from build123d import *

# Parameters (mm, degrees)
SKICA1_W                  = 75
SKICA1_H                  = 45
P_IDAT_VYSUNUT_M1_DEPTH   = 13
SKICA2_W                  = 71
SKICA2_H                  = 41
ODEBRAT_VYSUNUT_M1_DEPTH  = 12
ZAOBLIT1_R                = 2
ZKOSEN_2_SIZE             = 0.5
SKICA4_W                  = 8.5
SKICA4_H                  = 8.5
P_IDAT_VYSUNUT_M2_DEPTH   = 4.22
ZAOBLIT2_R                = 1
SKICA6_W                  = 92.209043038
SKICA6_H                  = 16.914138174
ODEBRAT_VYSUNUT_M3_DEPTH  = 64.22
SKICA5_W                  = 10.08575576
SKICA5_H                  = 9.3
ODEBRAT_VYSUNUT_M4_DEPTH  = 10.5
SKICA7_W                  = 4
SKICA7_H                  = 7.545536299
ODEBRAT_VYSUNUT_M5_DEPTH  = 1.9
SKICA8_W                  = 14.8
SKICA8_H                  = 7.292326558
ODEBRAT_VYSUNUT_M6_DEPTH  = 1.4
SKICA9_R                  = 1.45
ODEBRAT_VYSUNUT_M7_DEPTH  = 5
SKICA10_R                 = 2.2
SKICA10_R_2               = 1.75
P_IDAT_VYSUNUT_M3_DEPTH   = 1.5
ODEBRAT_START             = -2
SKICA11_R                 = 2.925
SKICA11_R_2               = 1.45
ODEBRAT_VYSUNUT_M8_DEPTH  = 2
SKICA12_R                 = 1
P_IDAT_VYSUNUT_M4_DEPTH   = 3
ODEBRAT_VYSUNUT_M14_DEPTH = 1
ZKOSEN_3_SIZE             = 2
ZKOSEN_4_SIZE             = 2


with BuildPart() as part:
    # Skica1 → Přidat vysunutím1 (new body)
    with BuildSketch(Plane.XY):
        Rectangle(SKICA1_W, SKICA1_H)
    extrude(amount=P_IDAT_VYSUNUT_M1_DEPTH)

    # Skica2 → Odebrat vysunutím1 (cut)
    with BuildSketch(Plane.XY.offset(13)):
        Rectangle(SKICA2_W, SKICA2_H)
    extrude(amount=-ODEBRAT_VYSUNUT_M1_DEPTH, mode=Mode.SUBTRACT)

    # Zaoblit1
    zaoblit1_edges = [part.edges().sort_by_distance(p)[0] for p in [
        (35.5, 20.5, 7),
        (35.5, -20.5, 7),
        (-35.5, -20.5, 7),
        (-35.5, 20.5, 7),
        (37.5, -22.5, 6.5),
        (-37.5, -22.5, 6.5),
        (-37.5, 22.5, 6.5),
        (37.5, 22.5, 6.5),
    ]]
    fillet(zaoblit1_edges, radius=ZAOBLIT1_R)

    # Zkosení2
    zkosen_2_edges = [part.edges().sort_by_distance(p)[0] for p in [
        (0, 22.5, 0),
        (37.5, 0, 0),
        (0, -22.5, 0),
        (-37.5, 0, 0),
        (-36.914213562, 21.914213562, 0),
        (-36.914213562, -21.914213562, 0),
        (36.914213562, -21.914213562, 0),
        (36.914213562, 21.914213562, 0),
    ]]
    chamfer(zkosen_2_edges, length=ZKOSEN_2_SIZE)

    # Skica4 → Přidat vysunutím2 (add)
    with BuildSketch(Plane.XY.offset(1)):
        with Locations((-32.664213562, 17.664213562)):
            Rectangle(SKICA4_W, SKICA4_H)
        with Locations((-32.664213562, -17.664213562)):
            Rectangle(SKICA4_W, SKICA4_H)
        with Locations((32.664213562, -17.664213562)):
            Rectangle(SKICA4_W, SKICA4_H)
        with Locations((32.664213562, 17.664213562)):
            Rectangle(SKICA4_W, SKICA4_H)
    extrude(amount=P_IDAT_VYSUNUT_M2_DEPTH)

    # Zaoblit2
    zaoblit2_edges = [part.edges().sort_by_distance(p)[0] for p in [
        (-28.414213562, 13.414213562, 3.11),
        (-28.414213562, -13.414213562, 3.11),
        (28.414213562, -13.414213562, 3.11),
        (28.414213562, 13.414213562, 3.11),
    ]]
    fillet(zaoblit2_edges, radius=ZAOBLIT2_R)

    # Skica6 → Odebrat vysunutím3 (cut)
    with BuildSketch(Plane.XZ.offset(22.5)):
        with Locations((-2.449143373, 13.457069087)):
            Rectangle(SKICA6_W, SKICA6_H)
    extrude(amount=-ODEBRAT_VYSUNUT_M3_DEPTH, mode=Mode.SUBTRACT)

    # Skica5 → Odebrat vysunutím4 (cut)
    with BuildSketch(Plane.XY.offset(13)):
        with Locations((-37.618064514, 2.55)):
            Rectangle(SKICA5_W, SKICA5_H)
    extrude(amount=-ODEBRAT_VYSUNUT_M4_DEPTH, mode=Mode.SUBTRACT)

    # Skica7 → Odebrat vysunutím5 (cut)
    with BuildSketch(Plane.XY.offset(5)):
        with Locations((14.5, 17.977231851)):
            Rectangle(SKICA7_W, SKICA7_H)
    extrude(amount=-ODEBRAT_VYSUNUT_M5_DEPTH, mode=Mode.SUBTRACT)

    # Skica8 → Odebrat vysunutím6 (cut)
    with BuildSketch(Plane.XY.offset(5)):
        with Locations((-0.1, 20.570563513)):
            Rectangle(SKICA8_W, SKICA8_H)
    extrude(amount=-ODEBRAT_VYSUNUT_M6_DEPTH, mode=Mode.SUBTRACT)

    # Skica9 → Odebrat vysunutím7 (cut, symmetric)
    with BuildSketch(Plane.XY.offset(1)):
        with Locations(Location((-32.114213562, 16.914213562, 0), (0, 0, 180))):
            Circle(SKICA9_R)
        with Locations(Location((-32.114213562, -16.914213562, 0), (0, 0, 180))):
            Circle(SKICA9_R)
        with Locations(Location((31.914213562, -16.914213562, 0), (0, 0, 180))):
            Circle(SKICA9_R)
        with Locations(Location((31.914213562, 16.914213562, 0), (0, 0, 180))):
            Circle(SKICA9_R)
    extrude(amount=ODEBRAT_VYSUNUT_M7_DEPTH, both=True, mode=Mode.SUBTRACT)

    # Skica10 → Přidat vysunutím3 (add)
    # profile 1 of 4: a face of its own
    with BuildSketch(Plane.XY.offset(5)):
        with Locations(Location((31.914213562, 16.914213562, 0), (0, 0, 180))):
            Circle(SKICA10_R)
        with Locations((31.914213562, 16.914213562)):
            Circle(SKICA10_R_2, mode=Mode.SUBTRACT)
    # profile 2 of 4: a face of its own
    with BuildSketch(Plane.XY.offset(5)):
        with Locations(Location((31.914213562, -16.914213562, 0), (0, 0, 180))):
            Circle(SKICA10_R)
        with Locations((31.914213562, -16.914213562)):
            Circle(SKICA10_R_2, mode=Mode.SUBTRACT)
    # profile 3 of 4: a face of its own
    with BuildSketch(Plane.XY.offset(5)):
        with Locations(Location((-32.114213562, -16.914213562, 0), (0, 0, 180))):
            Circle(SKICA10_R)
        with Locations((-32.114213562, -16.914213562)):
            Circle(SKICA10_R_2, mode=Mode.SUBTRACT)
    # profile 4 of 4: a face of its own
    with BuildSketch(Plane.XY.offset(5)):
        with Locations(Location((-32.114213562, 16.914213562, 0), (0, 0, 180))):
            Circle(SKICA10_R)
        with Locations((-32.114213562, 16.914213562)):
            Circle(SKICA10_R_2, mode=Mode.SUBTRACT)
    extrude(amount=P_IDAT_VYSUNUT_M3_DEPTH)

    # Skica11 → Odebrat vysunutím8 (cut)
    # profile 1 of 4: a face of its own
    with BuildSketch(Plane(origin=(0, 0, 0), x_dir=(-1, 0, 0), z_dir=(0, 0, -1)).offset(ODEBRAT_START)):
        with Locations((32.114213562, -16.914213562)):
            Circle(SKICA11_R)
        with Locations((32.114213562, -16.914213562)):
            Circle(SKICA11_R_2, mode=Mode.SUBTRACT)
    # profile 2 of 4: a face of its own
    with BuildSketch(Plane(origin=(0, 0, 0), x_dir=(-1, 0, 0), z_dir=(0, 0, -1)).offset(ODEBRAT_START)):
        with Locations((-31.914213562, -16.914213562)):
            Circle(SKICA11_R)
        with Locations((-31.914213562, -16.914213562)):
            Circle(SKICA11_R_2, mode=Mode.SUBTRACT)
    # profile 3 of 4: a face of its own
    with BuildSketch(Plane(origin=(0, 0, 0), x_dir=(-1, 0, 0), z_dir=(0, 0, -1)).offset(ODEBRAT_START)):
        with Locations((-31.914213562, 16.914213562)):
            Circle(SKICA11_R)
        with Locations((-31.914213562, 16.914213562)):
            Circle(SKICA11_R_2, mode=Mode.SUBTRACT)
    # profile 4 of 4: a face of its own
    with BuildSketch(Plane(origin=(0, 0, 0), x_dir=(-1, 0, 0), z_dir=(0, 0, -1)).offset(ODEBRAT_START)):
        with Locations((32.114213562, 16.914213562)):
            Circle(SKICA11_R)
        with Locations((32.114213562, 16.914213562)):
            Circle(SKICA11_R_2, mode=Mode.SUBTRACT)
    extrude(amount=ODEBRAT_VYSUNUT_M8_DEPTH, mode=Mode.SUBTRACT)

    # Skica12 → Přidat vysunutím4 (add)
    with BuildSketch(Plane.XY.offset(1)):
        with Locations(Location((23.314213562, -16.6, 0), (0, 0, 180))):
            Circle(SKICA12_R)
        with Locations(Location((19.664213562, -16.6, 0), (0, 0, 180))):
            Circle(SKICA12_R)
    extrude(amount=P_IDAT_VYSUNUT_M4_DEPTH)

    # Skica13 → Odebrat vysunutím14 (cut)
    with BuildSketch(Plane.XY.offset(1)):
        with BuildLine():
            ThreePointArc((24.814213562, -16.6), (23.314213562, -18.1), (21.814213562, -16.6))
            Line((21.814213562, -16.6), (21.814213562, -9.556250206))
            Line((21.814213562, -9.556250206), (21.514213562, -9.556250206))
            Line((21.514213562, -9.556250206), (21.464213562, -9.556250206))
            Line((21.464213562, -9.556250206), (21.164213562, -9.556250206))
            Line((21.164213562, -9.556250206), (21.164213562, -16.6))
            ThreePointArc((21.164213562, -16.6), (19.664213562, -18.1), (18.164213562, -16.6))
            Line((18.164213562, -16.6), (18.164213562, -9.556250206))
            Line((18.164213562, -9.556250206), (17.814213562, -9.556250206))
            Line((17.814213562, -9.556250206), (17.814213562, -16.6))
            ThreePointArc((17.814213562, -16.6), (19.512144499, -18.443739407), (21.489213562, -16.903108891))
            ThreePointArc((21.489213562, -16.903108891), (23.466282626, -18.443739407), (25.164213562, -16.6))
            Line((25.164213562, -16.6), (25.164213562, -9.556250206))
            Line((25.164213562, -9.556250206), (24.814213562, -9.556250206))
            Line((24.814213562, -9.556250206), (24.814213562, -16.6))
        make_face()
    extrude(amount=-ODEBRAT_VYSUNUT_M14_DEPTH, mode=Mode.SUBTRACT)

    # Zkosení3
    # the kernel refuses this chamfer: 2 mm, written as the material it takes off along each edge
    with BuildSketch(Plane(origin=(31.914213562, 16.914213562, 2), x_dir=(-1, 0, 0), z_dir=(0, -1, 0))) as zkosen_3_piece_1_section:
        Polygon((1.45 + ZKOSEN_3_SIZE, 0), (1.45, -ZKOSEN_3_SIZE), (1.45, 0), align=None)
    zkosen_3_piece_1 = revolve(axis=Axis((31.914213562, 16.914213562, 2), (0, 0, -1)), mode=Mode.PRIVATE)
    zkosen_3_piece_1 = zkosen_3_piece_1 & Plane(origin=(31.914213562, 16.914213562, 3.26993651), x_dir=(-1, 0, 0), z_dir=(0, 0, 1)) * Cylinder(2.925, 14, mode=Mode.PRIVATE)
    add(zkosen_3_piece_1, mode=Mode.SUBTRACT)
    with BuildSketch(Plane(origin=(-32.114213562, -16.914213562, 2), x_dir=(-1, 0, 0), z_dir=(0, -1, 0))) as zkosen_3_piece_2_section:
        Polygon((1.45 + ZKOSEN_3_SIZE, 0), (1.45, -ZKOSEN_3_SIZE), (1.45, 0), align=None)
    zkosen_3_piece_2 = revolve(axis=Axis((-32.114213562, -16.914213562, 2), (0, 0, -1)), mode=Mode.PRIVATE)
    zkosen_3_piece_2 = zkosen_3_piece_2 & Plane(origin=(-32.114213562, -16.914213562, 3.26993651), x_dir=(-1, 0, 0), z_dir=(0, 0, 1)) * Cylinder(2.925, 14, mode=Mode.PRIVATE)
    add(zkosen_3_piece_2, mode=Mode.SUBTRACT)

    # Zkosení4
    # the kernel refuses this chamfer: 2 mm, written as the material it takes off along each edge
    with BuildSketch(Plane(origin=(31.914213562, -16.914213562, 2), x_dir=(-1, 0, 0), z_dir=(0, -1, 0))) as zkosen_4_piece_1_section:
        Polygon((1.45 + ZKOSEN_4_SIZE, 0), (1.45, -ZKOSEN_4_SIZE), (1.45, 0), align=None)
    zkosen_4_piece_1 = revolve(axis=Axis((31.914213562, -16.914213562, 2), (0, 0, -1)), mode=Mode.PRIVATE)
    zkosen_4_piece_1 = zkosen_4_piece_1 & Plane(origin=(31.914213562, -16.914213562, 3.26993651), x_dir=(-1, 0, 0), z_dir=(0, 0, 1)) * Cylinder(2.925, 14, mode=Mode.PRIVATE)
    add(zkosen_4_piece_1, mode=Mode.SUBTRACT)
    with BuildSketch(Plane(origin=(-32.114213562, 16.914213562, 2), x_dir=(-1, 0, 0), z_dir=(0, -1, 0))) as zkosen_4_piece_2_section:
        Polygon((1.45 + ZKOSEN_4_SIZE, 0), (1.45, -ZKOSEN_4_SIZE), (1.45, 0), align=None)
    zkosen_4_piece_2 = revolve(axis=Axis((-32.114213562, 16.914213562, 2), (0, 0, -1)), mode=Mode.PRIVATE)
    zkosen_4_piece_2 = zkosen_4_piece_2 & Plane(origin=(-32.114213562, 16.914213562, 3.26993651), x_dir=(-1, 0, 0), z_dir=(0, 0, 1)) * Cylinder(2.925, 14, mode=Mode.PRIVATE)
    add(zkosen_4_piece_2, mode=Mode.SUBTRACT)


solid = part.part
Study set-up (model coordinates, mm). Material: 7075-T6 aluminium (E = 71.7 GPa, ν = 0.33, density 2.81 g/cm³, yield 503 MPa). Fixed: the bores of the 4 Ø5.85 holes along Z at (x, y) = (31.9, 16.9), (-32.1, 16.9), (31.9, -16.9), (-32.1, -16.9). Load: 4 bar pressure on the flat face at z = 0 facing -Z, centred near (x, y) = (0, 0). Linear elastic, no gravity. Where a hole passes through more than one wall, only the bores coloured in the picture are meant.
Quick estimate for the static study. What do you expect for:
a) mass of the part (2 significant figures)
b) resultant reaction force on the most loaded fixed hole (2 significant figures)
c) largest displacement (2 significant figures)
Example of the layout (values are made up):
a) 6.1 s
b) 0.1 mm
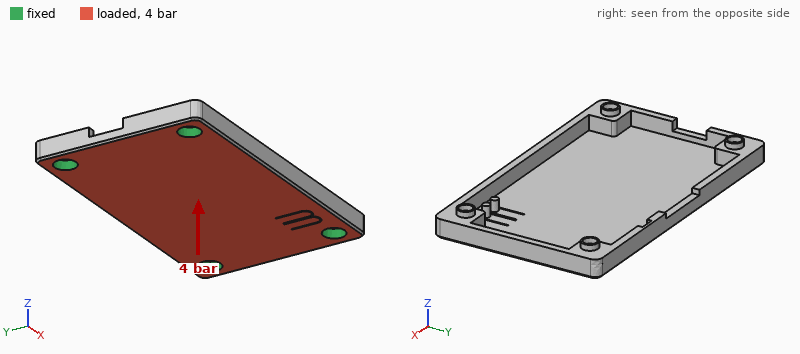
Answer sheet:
a) 16 g
b) 390 N
c) 0.87 mm
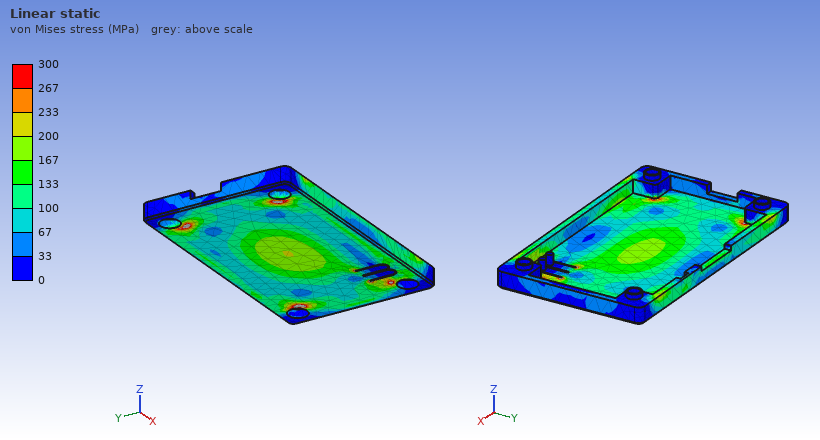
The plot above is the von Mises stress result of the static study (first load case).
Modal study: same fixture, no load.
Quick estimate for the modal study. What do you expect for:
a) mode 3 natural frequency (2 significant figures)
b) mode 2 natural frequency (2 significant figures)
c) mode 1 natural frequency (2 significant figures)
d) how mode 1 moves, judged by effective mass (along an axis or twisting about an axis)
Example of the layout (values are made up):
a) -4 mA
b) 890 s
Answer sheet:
a) 4900 Hz
b) 4500 Hz
c) 2600 Hz
d) along Z
